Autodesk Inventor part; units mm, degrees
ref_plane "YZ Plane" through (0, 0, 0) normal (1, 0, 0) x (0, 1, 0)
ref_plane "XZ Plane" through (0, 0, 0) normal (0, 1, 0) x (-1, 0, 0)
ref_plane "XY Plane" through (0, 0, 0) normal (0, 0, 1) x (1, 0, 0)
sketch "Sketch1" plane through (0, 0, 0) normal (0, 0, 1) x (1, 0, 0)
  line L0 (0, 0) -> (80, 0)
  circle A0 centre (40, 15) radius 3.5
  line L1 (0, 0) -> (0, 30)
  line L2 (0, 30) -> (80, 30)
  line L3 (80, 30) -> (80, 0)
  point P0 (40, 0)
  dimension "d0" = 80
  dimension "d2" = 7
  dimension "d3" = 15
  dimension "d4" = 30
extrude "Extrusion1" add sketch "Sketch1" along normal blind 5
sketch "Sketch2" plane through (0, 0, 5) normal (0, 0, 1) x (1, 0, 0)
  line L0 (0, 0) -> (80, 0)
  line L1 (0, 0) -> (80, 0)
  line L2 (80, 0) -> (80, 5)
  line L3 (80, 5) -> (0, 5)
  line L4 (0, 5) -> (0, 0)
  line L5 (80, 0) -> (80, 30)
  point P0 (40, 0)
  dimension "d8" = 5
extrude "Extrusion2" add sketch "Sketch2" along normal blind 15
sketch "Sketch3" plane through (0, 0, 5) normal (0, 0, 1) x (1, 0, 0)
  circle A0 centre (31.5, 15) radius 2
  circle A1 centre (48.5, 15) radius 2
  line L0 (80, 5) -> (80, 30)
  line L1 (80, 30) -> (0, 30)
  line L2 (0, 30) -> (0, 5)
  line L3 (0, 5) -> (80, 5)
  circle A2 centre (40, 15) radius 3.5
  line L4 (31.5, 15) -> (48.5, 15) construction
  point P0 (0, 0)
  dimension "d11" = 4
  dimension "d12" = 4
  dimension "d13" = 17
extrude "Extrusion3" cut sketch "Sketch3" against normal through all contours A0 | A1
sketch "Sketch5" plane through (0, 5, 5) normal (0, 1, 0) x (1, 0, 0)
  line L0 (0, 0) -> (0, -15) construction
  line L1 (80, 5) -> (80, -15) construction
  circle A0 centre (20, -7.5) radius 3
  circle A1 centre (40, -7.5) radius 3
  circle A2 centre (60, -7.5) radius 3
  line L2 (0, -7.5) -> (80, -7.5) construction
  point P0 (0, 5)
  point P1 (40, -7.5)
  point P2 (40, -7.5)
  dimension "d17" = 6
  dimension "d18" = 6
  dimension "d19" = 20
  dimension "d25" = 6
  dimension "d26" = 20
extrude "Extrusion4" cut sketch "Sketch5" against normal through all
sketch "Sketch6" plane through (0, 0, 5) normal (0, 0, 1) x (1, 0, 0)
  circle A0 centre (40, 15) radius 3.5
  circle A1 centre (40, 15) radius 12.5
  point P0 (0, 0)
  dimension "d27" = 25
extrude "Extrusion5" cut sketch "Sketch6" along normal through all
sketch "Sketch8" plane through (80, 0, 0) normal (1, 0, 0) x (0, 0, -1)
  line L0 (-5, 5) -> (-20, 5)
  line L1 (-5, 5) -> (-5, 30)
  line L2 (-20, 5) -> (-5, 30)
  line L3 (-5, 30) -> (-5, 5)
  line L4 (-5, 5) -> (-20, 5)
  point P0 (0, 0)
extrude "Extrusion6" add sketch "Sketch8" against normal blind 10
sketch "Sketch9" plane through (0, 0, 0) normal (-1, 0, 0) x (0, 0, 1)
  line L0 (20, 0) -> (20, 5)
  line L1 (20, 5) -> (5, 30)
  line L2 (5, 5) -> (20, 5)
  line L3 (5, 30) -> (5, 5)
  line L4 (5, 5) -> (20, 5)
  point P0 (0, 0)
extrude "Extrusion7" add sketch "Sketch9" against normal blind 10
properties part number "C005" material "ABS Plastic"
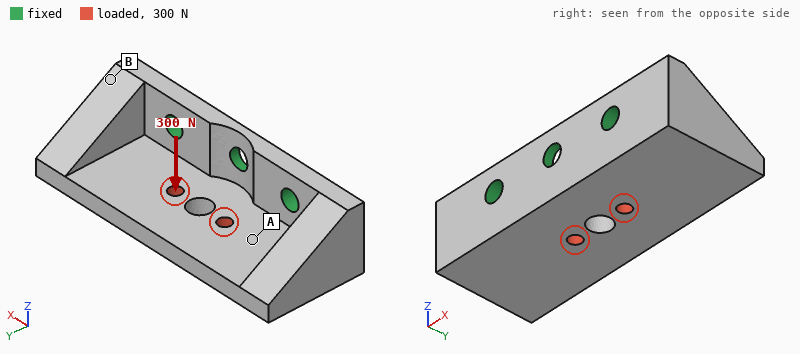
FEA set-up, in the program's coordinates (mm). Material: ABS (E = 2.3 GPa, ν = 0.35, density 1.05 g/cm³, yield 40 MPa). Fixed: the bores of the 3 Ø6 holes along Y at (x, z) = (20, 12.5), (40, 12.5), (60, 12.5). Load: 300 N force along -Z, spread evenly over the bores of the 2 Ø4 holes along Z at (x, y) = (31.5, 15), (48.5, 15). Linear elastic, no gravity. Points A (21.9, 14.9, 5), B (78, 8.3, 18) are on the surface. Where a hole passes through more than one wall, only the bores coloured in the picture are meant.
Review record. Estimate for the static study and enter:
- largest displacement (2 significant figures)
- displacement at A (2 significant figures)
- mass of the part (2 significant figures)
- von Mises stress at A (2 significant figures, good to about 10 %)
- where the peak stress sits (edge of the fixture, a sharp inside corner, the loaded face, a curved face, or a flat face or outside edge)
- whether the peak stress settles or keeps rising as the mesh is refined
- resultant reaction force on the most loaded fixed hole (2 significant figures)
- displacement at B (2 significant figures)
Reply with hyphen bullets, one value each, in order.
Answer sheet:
- 0.72 mm
- 0.26 mm
- 22 g
- 4.4 MPa
- edge of the fixture
- keeps rising
- 120 N
- 0.13 mm
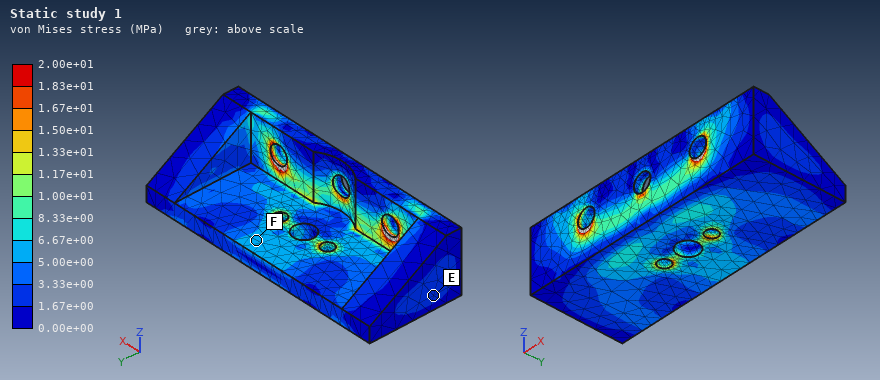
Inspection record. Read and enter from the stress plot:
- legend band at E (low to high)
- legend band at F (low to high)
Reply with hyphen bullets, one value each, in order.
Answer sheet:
- 1.67e+00 to 3.33e+00 MPa
- 5.00e+00 to 6.67e+00 MPa
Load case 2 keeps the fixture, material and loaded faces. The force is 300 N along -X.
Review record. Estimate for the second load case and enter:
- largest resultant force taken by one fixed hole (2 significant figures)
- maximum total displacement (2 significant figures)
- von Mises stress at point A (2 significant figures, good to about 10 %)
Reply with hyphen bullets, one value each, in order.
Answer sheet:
- 150 N
- 0.14 mm
- 2.3 MPa
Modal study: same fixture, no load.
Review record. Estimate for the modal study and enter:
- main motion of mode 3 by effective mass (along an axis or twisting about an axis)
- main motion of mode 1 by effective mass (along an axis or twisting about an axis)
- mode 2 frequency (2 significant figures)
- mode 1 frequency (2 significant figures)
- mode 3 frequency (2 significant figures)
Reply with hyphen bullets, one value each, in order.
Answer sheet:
- along X
- along Z
- 1400 Hz
- 1200 Hz
- 2500 Hz
